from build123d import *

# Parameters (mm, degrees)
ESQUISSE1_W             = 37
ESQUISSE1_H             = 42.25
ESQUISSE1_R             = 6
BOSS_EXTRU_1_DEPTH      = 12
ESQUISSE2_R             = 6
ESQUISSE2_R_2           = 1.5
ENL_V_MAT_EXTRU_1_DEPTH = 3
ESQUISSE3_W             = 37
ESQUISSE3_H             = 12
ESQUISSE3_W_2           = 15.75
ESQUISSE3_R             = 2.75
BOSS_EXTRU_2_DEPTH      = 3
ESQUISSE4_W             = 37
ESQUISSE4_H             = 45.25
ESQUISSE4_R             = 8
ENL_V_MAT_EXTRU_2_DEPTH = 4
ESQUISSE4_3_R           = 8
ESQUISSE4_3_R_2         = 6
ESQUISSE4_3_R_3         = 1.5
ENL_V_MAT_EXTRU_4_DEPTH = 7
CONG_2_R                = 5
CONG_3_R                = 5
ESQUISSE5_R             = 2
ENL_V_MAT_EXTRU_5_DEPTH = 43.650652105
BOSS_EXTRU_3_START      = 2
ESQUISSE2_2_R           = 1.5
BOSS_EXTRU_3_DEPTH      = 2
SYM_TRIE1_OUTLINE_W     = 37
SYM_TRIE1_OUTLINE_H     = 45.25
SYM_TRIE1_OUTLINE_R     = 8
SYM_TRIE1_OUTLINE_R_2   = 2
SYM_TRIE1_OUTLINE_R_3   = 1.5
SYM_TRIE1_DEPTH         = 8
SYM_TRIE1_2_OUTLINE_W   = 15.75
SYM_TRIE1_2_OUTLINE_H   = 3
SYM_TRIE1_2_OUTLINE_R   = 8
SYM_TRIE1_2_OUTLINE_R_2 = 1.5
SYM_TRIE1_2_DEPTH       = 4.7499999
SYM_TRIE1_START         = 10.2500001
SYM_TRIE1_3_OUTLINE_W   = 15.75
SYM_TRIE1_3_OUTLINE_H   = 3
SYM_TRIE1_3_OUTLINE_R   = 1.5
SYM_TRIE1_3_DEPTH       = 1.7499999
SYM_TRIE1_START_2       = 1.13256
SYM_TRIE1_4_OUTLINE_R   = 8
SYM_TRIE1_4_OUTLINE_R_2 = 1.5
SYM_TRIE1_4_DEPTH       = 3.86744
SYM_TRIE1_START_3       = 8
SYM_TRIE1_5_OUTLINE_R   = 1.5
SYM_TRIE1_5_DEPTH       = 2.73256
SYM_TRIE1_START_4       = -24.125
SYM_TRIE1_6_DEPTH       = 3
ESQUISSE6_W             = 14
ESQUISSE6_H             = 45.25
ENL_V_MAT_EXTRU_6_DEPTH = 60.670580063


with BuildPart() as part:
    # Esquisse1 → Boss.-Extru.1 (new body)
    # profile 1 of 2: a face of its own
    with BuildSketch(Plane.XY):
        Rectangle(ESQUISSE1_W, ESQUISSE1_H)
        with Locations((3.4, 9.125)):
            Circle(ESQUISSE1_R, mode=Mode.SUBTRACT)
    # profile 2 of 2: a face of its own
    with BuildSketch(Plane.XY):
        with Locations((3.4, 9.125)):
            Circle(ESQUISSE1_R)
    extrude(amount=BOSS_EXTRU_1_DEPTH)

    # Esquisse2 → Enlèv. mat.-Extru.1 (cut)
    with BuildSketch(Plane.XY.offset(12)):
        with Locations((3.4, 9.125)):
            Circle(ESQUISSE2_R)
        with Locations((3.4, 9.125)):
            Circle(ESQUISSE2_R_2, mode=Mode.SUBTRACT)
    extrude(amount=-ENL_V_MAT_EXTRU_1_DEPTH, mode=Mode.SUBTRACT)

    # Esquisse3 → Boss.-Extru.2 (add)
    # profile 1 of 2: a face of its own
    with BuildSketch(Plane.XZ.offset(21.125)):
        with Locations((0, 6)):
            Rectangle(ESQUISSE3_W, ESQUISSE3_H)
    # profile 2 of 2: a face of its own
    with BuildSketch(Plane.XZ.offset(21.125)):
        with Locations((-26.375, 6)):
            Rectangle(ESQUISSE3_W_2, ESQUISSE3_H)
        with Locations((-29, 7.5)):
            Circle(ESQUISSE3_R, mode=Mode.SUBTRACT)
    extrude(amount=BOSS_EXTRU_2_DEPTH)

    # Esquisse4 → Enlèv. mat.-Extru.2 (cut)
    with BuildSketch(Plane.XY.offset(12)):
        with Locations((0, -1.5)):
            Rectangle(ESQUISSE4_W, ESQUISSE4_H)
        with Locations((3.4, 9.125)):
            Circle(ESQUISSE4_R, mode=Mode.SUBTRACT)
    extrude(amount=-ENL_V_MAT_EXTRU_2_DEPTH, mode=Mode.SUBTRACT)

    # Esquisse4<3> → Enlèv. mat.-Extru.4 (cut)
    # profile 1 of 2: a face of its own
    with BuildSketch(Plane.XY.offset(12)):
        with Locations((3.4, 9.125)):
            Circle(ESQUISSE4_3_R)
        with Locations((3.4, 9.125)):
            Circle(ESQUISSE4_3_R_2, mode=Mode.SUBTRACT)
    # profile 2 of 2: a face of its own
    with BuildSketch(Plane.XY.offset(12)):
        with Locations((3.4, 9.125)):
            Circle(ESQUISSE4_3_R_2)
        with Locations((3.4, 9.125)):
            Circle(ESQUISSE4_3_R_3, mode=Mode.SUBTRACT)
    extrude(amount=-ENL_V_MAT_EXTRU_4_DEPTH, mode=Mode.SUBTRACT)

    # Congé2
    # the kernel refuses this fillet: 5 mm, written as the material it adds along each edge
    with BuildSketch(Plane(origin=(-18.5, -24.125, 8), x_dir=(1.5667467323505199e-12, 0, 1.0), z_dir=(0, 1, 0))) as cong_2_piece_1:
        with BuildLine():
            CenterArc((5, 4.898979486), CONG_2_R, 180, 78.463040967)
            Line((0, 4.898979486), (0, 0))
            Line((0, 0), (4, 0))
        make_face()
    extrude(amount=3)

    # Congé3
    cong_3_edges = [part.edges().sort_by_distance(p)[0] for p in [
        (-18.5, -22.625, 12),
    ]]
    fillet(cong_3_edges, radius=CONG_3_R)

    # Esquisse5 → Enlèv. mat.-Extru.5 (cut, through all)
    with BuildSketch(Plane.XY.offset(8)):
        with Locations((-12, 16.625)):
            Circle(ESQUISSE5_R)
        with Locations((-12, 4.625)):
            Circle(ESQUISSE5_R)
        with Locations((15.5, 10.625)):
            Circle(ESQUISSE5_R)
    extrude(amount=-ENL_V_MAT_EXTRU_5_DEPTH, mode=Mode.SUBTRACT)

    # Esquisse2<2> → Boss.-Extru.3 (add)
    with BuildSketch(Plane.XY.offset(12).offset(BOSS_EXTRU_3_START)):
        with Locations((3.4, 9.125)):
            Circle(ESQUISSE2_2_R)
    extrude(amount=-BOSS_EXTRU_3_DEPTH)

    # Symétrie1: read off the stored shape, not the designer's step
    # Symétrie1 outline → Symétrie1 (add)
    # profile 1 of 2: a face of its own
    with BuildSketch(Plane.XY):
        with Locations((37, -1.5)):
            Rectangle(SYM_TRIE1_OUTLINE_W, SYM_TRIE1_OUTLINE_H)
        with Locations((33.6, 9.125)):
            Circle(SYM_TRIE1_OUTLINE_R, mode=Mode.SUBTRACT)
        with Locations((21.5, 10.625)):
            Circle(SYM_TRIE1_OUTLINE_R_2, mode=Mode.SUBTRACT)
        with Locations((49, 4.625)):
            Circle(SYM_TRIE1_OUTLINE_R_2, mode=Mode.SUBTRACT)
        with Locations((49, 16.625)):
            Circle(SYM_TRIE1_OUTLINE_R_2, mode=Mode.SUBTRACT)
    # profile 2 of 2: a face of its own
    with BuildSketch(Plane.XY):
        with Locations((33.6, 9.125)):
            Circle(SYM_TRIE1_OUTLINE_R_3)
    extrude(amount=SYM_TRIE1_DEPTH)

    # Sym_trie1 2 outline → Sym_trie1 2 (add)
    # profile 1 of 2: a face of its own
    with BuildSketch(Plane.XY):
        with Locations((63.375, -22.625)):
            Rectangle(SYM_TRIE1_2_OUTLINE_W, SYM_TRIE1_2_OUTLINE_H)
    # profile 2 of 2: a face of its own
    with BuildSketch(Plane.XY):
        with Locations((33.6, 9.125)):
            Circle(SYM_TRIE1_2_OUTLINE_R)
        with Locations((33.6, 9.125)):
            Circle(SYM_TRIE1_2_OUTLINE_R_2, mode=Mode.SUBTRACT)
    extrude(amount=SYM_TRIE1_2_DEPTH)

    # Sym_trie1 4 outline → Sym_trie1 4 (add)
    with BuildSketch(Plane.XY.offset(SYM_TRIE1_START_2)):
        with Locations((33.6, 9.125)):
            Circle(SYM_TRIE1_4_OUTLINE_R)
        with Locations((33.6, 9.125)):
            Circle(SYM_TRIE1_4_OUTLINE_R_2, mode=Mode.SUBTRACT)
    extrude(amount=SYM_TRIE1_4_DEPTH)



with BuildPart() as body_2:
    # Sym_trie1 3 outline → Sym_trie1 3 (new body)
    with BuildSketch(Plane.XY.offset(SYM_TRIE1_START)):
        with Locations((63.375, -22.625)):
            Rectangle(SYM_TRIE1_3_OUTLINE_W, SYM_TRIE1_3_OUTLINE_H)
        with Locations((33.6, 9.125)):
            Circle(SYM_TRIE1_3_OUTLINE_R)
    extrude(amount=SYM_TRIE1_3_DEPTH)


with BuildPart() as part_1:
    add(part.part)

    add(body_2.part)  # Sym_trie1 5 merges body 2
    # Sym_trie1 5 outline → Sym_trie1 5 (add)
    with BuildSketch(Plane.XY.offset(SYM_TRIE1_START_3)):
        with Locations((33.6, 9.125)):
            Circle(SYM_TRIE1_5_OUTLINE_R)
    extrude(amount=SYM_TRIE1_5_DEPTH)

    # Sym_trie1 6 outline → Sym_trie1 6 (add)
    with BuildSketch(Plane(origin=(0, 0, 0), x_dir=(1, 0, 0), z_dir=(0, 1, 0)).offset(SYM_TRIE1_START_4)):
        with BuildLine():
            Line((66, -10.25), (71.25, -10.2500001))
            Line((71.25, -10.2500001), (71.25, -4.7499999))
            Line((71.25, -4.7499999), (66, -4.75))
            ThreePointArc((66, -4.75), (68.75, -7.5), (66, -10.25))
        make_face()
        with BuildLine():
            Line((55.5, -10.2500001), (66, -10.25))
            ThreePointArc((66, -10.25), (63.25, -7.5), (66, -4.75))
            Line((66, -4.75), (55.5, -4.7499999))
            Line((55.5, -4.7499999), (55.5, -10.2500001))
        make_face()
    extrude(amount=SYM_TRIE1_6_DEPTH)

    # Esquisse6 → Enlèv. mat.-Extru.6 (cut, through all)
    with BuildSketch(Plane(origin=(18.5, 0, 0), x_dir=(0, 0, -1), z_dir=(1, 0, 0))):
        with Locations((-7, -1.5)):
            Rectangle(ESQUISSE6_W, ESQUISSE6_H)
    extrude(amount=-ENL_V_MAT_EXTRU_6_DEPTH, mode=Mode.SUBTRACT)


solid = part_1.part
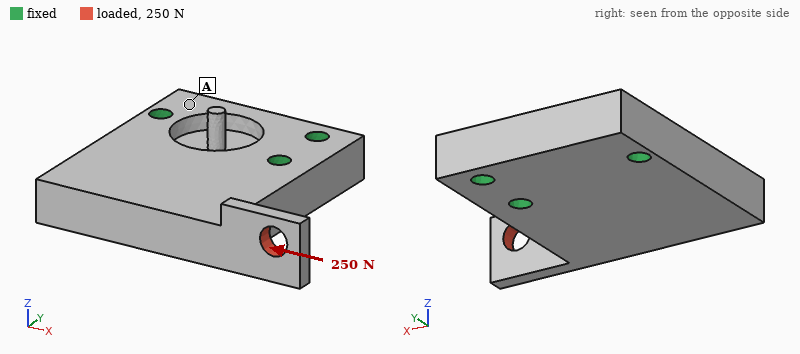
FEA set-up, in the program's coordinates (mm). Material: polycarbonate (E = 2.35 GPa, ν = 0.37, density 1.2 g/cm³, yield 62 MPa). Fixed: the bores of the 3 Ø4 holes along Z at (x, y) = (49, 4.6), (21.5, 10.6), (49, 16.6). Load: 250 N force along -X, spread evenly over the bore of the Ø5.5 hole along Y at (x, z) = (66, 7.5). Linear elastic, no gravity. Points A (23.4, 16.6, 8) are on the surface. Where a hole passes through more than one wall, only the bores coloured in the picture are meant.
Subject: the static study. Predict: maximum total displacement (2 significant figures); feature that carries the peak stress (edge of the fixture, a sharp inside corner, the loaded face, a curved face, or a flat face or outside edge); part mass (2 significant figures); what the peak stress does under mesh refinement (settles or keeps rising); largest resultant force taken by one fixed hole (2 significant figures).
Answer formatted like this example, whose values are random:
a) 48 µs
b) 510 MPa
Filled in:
a) 0.71 mm
b) a sharp inside corner
c) 16 g
d) keeps rising
e) 280 N
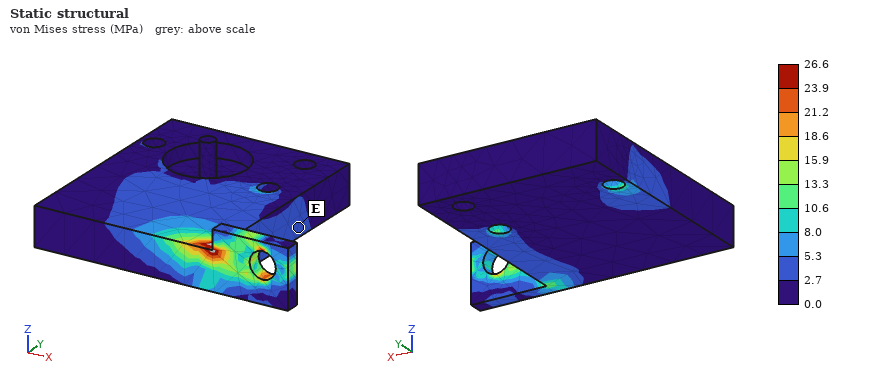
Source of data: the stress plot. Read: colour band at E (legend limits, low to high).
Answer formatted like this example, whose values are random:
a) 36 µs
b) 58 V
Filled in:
a) 2.7 to 5.3 MPa
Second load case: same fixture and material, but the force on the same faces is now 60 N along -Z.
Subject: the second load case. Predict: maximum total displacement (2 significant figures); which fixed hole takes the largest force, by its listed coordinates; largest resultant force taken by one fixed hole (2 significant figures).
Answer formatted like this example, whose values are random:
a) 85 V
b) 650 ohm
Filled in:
a) 0.80 mm
b) (49, 4.6)
c) 120 N
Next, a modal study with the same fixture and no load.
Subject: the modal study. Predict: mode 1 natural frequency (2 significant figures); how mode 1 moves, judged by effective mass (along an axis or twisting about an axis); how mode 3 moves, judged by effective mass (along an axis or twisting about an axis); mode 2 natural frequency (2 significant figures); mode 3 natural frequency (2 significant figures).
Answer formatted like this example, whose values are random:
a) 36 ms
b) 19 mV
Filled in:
a) 1500 Hz
b) along Z
c) twisting about Y
d) 2100 Hz
e) 2200 Hz
